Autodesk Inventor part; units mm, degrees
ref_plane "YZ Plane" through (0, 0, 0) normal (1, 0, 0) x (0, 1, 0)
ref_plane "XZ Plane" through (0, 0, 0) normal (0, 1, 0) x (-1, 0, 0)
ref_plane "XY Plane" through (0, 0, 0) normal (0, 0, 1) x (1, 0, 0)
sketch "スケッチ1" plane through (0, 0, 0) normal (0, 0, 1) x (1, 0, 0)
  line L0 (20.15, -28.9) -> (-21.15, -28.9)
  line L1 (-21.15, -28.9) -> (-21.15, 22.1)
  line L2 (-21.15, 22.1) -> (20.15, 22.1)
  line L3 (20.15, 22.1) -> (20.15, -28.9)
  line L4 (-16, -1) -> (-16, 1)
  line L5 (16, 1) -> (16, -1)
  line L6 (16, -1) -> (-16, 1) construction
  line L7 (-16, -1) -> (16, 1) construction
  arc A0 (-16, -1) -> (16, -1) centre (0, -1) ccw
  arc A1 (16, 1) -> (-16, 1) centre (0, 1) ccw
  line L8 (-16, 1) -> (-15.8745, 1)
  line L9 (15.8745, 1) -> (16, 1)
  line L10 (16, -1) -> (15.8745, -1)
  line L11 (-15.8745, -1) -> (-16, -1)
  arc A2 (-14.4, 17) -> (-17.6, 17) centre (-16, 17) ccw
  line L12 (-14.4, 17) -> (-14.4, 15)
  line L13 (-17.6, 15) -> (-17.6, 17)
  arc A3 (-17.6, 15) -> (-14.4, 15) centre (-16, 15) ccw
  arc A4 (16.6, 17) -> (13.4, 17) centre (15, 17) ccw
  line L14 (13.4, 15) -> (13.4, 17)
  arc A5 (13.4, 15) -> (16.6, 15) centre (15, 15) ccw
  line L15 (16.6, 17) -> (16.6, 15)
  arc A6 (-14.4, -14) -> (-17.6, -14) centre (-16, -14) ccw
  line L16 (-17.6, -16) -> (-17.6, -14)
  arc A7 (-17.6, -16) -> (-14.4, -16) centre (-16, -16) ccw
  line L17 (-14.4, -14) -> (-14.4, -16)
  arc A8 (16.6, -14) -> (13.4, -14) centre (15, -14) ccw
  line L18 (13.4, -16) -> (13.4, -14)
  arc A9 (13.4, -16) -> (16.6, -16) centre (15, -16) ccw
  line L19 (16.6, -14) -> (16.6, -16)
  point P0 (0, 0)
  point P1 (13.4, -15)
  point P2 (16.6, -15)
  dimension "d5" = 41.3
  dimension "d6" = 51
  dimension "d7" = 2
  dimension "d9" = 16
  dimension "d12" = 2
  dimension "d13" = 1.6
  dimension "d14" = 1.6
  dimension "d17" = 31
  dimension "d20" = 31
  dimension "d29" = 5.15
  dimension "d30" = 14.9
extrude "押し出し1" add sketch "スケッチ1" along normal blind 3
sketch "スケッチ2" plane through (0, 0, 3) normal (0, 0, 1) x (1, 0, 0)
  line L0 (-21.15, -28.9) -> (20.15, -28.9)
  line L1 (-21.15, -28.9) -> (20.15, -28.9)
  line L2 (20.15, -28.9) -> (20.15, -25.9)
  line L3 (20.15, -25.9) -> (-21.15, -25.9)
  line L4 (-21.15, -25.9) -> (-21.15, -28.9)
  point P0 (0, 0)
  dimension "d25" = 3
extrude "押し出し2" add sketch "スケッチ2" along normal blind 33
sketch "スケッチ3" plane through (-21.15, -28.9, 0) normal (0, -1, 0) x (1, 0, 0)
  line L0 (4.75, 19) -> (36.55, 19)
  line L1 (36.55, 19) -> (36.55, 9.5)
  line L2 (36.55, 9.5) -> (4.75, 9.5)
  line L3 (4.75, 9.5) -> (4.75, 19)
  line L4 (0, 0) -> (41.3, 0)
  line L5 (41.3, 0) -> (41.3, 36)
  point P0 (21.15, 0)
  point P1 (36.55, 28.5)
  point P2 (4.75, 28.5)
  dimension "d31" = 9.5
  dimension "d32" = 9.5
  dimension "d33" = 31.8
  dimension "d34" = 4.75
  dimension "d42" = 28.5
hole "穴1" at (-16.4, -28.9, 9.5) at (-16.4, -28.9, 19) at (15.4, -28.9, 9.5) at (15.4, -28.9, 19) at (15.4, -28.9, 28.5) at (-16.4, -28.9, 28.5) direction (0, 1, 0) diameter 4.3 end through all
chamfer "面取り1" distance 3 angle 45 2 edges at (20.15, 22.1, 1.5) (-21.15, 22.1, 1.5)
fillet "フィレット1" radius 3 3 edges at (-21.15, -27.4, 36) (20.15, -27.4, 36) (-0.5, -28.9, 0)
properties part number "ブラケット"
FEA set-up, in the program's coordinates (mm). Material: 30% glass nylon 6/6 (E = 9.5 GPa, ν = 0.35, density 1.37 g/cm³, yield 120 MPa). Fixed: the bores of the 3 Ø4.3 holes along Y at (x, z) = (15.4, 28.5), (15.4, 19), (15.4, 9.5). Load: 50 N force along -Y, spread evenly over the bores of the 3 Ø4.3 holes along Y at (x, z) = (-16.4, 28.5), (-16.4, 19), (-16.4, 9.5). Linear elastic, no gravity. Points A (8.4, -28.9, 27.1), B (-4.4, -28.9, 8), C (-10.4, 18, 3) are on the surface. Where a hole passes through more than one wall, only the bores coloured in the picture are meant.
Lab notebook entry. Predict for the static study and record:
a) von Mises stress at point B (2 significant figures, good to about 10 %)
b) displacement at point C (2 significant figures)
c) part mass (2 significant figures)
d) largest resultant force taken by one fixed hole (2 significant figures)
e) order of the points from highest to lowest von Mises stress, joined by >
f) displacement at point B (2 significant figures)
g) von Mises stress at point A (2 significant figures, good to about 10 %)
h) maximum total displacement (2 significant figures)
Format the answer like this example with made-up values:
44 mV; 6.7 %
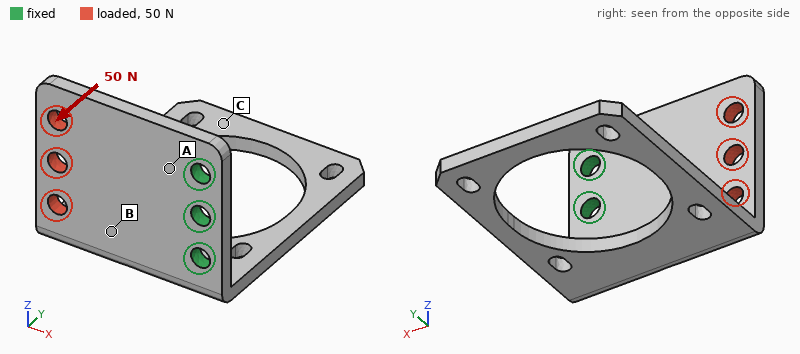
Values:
7.2 MPa; 0.48 mm; 9.9 g; 21 N; A > B > C; 0.17 mm; 15 MPa; 0.55 mm
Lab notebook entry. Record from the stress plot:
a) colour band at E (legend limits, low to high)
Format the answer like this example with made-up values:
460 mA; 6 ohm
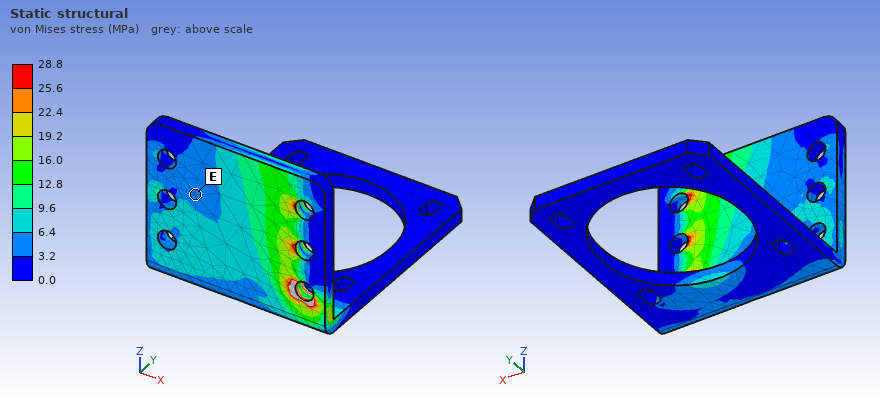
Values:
3.2 to 6.4 MPa
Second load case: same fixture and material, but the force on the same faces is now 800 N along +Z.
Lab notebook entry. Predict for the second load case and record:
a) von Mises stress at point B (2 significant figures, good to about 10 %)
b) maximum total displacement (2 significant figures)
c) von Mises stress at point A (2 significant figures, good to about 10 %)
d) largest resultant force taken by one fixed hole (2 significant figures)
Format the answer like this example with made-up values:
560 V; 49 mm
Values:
15 MPa; 0.25 mm; 30 MPa; 1.1 kN
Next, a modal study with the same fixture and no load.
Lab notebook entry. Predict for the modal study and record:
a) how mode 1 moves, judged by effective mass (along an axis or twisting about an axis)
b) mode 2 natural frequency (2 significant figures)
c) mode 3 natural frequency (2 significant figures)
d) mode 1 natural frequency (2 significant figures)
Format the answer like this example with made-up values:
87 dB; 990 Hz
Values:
along Z; 650 Hz; 1000 Hz; 390 Hz
